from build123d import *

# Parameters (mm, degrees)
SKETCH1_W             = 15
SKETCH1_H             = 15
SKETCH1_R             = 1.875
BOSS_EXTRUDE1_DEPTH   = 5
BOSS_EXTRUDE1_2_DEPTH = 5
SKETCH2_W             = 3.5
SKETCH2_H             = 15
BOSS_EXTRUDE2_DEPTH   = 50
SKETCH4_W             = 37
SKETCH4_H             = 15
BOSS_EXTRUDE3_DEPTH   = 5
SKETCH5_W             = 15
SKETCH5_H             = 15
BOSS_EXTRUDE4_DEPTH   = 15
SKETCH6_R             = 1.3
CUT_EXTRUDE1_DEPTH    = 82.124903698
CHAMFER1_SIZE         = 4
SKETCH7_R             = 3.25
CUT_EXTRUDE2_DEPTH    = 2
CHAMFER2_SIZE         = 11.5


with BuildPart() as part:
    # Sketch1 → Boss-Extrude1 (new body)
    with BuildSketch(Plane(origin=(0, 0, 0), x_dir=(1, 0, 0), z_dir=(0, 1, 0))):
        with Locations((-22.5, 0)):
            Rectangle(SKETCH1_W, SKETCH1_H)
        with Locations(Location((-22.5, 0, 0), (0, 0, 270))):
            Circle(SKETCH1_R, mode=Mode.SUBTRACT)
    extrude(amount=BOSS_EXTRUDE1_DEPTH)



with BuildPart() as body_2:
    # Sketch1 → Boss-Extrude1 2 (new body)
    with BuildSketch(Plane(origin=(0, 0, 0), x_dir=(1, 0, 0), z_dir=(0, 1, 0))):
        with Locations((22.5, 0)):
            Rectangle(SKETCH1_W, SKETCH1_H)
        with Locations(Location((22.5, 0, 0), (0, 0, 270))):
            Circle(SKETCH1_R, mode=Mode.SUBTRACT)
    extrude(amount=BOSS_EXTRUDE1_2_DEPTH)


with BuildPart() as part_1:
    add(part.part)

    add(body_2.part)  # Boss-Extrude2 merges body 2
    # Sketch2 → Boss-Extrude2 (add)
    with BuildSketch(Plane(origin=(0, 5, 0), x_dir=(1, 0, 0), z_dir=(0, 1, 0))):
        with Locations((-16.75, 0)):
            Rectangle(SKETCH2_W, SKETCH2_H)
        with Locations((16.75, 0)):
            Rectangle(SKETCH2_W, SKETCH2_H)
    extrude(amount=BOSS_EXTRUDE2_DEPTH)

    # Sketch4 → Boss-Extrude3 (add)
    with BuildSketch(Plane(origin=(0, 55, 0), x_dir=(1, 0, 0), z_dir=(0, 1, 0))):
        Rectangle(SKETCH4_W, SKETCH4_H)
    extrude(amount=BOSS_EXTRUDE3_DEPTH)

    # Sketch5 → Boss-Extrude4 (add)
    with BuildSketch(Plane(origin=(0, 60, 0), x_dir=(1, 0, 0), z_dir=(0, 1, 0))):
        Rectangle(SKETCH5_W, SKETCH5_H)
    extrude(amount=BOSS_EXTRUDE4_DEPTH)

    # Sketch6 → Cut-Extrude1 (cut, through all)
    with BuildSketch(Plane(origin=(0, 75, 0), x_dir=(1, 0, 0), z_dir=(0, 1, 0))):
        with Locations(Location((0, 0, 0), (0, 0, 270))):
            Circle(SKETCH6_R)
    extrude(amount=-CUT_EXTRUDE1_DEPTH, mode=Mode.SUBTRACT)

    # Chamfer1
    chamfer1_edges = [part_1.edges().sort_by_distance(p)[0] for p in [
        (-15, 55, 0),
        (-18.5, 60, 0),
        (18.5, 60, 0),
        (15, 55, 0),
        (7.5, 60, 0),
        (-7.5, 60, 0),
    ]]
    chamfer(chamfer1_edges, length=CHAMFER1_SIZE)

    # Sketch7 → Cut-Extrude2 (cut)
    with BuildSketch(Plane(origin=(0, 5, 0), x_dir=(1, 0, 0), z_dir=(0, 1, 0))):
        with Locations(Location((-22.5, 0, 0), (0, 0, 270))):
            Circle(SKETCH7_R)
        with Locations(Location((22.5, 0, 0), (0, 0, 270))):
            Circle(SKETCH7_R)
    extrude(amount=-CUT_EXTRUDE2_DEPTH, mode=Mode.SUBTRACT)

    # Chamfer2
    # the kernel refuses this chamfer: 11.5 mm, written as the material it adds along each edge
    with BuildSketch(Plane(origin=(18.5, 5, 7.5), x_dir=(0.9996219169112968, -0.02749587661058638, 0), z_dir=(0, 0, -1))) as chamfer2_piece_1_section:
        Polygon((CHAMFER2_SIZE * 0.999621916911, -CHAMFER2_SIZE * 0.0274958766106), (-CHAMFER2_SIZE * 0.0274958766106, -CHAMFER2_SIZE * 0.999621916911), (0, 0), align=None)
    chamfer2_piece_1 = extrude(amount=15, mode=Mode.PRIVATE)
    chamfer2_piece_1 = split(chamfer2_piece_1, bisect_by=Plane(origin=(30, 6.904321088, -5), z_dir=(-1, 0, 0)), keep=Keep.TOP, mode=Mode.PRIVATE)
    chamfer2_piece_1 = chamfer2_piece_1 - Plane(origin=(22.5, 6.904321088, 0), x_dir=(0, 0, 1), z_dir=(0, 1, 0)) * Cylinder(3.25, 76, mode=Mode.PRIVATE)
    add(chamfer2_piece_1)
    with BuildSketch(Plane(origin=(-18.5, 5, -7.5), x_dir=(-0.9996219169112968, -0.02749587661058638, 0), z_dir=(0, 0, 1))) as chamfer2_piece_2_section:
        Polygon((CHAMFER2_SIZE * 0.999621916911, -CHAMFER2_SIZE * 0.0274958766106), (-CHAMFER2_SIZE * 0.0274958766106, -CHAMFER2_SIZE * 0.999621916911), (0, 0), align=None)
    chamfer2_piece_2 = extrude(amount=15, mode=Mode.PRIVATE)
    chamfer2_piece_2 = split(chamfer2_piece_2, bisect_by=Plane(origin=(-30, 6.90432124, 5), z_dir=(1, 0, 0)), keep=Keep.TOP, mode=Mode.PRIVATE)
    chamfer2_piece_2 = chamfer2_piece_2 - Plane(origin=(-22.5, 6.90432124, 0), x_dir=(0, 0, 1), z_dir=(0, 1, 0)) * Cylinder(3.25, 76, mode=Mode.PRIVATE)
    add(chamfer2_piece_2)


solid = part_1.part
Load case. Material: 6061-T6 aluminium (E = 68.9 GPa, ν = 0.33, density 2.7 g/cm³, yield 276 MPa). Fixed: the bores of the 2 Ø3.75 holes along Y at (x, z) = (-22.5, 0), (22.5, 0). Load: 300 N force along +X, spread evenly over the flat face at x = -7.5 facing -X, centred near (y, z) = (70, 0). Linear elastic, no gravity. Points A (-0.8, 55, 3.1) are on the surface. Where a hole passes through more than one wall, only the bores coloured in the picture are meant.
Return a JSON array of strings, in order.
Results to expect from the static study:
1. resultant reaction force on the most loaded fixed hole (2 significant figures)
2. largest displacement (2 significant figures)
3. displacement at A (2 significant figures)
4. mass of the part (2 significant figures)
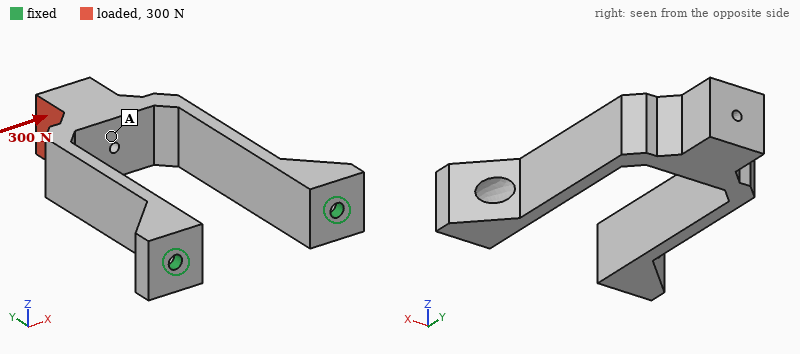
["360 N", "0.26 mm", "0.26 mm", "41 g"]
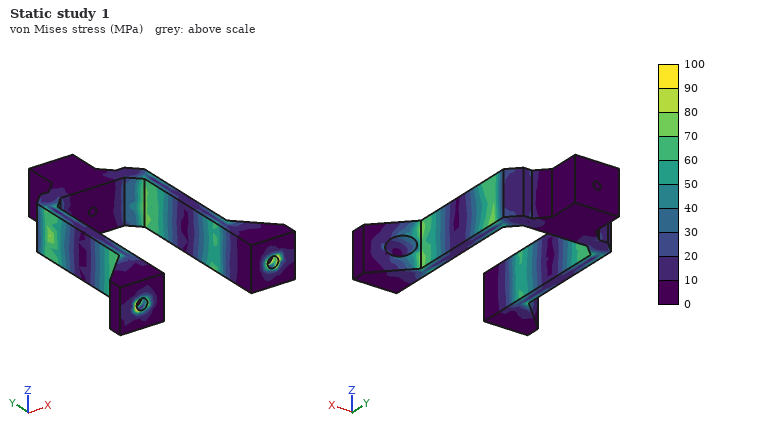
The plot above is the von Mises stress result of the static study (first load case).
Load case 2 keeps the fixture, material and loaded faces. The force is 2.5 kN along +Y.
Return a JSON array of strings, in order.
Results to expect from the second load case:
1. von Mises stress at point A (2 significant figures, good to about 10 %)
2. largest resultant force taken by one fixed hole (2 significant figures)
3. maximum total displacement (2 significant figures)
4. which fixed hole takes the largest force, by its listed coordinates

["46 MPa", "1.8 kN", "82 µm", "(-22.5, 0)"]
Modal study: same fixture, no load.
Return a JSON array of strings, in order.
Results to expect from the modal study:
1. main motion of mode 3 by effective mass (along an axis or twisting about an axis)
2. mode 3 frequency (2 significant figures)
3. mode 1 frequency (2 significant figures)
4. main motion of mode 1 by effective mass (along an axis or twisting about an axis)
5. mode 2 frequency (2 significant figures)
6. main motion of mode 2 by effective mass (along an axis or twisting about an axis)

["twisting about Y", "3000 Hz", "1000 Hz", "along Z", "1200 Hz", "along X"]
